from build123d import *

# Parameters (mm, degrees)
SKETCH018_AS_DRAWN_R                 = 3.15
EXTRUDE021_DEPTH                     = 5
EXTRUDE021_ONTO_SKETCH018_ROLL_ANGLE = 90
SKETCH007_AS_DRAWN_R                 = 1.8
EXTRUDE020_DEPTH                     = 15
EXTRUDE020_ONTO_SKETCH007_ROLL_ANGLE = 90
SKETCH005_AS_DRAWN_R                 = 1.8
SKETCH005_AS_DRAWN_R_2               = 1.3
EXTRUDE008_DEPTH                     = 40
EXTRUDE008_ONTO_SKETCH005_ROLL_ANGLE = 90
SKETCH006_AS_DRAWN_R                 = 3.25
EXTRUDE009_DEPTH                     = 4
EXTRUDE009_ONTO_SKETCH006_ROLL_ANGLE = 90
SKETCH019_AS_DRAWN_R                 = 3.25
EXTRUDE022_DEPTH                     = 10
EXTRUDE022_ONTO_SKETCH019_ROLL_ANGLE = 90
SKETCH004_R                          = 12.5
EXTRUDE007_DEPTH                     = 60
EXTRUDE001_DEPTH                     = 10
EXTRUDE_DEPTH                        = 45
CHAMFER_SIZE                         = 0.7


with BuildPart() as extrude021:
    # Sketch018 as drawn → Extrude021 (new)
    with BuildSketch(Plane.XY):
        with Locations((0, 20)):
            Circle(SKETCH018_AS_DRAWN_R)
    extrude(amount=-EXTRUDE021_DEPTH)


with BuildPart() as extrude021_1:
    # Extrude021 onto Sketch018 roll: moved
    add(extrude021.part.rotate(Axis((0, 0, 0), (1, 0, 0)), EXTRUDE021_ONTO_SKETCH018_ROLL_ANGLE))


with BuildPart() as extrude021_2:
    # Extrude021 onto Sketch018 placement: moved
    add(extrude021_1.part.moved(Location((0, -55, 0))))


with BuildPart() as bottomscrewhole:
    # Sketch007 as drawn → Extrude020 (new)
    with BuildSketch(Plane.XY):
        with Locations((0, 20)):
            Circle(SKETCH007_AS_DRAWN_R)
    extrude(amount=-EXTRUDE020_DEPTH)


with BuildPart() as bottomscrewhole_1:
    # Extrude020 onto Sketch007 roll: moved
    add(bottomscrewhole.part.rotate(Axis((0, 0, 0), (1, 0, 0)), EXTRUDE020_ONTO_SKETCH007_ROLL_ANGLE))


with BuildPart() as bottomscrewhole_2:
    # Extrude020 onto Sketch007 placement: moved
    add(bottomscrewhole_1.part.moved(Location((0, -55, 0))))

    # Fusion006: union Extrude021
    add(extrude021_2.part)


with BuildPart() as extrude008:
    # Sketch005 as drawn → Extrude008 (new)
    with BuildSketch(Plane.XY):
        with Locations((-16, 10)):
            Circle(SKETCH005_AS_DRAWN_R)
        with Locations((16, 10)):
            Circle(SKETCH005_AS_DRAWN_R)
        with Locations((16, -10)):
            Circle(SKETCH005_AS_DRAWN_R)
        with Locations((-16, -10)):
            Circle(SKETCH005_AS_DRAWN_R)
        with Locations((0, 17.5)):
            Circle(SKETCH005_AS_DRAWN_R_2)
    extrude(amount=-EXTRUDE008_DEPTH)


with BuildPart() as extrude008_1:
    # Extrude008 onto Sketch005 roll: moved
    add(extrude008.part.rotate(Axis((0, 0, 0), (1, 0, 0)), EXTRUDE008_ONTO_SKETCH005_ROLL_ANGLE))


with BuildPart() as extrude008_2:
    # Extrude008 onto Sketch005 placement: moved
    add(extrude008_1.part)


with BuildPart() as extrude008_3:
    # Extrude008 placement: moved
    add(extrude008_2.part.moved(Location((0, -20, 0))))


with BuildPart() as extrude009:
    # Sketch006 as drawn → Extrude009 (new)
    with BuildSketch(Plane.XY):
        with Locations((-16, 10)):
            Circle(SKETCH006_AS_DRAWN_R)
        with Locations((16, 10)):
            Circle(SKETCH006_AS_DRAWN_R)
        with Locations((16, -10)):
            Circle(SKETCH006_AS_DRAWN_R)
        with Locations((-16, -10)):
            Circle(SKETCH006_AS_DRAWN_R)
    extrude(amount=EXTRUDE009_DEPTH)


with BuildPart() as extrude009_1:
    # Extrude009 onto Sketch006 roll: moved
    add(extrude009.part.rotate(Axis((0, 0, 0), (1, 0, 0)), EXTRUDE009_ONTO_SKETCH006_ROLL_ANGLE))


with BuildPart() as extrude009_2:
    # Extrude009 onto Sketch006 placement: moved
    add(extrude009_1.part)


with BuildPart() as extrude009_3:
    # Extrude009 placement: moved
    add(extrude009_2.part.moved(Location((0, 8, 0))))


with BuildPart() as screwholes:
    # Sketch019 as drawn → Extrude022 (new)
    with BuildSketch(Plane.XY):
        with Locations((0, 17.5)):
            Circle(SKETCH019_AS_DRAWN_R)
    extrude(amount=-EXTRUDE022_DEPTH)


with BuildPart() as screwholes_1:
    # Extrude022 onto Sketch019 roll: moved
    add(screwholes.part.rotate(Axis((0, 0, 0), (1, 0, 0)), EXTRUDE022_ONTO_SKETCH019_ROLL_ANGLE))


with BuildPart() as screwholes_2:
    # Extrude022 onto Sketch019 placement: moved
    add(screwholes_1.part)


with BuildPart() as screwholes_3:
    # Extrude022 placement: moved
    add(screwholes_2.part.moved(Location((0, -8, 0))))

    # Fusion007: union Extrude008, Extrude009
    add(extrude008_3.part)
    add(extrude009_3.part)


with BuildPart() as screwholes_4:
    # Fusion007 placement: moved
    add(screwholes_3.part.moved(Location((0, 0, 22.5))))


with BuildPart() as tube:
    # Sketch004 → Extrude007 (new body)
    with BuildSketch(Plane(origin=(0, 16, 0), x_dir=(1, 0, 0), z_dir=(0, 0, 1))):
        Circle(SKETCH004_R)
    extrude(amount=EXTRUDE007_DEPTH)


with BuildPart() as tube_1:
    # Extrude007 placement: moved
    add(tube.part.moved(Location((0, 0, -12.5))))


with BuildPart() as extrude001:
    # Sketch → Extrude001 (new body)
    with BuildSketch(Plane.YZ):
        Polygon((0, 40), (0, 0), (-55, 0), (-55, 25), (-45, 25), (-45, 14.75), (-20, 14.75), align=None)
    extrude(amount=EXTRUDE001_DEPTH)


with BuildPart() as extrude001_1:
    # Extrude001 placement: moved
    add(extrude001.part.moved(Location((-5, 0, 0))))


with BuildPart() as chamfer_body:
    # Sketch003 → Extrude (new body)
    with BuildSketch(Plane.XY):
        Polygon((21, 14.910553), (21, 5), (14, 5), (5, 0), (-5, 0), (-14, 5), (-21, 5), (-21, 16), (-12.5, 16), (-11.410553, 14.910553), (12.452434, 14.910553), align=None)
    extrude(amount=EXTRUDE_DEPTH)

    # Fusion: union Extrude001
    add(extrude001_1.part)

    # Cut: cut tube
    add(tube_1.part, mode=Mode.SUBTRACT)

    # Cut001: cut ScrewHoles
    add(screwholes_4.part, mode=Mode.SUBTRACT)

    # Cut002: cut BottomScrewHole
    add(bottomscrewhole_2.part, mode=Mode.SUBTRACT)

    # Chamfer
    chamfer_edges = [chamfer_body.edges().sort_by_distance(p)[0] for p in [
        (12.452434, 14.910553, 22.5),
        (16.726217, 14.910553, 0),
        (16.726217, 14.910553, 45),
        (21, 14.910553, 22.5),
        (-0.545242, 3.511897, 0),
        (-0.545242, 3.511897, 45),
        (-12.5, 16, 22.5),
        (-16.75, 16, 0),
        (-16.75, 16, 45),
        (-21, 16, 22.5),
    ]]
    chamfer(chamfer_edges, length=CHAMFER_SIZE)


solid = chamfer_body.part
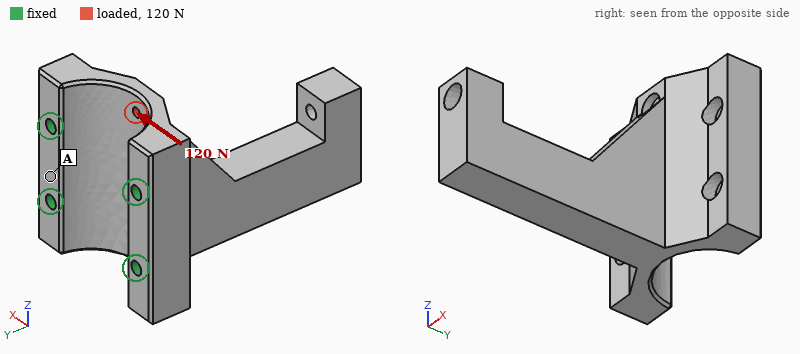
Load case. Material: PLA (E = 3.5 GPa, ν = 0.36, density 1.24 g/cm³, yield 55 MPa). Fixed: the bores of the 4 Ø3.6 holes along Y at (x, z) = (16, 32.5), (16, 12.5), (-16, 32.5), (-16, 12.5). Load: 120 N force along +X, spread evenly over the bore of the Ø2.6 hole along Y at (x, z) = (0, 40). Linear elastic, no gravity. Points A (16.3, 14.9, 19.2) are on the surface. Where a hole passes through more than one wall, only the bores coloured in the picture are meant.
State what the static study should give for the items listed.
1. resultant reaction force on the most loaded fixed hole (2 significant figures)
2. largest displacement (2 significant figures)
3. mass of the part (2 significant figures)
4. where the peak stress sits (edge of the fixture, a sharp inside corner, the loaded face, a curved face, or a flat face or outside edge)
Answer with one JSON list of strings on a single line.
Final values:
["57 N", "22 µm", "30 g", "the loaded face"]
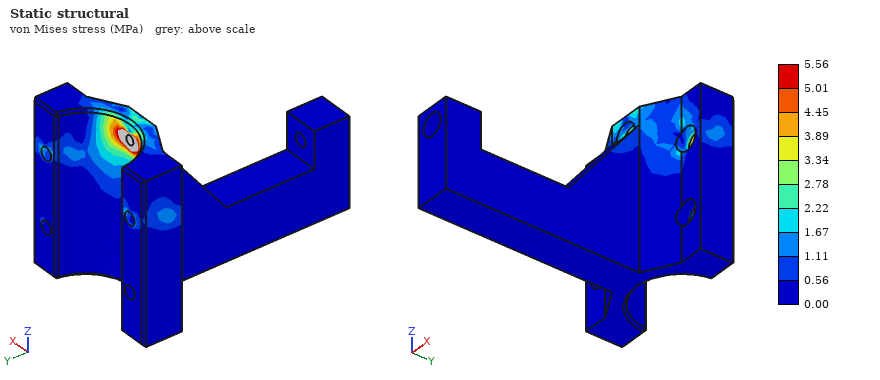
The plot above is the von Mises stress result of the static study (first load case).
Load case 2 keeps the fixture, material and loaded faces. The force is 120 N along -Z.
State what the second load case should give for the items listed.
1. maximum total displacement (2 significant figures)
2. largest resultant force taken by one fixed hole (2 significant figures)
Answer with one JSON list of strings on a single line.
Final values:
["22 µm", "42 N"]
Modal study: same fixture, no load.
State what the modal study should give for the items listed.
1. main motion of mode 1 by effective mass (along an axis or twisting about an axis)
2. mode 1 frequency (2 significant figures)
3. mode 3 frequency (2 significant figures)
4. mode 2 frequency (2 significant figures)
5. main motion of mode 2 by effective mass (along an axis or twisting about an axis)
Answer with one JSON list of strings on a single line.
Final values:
["along X", "720 Hz", "2900 Hz", "1200 Hz", "along Z"]
